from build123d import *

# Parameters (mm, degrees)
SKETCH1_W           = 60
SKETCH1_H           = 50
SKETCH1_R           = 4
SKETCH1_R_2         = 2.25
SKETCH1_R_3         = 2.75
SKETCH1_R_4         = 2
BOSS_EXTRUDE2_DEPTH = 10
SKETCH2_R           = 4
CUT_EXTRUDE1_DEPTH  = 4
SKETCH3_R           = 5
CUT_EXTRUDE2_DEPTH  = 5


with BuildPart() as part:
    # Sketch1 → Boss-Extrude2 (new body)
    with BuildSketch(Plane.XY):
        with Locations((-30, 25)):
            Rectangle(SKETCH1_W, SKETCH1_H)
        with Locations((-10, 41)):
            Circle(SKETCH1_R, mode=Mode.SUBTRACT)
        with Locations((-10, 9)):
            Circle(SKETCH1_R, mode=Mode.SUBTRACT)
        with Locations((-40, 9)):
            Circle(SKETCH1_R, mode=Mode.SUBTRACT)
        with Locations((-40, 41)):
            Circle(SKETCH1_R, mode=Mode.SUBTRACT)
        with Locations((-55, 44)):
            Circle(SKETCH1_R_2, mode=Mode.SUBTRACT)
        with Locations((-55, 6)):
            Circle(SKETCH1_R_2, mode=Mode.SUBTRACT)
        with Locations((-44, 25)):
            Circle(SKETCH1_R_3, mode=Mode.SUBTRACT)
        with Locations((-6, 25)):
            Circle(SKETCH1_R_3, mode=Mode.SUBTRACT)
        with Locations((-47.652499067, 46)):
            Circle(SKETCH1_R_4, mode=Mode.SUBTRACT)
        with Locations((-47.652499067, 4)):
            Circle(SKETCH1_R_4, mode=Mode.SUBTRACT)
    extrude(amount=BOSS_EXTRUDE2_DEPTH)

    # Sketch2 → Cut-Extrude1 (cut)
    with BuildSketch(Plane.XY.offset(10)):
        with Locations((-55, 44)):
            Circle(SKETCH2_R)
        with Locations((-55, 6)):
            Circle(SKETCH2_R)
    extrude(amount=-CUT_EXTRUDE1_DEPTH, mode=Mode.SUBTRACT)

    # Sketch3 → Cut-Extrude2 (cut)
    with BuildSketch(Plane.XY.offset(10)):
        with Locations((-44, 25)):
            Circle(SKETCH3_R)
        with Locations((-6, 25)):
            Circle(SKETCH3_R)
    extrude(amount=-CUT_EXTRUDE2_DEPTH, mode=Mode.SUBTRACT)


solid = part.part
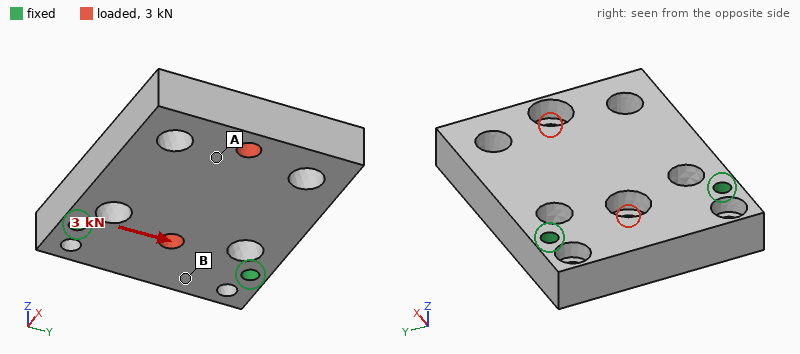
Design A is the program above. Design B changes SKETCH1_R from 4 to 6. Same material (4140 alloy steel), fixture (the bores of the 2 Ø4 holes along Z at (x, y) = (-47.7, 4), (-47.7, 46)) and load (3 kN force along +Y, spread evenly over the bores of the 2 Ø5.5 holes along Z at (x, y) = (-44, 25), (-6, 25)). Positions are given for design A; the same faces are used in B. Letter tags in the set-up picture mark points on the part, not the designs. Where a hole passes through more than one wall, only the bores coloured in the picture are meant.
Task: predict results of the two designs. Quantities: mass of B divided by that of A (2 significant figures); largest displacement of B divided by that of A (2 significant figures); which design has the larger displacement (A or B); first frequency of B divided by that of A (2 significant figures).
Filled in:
0.90
1.5
B
0.87
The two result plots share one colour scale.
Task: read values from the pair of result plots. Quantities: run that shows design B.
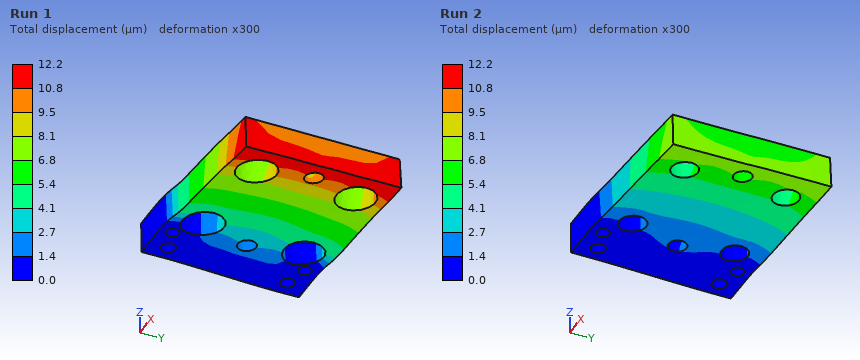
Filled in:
Run 1
